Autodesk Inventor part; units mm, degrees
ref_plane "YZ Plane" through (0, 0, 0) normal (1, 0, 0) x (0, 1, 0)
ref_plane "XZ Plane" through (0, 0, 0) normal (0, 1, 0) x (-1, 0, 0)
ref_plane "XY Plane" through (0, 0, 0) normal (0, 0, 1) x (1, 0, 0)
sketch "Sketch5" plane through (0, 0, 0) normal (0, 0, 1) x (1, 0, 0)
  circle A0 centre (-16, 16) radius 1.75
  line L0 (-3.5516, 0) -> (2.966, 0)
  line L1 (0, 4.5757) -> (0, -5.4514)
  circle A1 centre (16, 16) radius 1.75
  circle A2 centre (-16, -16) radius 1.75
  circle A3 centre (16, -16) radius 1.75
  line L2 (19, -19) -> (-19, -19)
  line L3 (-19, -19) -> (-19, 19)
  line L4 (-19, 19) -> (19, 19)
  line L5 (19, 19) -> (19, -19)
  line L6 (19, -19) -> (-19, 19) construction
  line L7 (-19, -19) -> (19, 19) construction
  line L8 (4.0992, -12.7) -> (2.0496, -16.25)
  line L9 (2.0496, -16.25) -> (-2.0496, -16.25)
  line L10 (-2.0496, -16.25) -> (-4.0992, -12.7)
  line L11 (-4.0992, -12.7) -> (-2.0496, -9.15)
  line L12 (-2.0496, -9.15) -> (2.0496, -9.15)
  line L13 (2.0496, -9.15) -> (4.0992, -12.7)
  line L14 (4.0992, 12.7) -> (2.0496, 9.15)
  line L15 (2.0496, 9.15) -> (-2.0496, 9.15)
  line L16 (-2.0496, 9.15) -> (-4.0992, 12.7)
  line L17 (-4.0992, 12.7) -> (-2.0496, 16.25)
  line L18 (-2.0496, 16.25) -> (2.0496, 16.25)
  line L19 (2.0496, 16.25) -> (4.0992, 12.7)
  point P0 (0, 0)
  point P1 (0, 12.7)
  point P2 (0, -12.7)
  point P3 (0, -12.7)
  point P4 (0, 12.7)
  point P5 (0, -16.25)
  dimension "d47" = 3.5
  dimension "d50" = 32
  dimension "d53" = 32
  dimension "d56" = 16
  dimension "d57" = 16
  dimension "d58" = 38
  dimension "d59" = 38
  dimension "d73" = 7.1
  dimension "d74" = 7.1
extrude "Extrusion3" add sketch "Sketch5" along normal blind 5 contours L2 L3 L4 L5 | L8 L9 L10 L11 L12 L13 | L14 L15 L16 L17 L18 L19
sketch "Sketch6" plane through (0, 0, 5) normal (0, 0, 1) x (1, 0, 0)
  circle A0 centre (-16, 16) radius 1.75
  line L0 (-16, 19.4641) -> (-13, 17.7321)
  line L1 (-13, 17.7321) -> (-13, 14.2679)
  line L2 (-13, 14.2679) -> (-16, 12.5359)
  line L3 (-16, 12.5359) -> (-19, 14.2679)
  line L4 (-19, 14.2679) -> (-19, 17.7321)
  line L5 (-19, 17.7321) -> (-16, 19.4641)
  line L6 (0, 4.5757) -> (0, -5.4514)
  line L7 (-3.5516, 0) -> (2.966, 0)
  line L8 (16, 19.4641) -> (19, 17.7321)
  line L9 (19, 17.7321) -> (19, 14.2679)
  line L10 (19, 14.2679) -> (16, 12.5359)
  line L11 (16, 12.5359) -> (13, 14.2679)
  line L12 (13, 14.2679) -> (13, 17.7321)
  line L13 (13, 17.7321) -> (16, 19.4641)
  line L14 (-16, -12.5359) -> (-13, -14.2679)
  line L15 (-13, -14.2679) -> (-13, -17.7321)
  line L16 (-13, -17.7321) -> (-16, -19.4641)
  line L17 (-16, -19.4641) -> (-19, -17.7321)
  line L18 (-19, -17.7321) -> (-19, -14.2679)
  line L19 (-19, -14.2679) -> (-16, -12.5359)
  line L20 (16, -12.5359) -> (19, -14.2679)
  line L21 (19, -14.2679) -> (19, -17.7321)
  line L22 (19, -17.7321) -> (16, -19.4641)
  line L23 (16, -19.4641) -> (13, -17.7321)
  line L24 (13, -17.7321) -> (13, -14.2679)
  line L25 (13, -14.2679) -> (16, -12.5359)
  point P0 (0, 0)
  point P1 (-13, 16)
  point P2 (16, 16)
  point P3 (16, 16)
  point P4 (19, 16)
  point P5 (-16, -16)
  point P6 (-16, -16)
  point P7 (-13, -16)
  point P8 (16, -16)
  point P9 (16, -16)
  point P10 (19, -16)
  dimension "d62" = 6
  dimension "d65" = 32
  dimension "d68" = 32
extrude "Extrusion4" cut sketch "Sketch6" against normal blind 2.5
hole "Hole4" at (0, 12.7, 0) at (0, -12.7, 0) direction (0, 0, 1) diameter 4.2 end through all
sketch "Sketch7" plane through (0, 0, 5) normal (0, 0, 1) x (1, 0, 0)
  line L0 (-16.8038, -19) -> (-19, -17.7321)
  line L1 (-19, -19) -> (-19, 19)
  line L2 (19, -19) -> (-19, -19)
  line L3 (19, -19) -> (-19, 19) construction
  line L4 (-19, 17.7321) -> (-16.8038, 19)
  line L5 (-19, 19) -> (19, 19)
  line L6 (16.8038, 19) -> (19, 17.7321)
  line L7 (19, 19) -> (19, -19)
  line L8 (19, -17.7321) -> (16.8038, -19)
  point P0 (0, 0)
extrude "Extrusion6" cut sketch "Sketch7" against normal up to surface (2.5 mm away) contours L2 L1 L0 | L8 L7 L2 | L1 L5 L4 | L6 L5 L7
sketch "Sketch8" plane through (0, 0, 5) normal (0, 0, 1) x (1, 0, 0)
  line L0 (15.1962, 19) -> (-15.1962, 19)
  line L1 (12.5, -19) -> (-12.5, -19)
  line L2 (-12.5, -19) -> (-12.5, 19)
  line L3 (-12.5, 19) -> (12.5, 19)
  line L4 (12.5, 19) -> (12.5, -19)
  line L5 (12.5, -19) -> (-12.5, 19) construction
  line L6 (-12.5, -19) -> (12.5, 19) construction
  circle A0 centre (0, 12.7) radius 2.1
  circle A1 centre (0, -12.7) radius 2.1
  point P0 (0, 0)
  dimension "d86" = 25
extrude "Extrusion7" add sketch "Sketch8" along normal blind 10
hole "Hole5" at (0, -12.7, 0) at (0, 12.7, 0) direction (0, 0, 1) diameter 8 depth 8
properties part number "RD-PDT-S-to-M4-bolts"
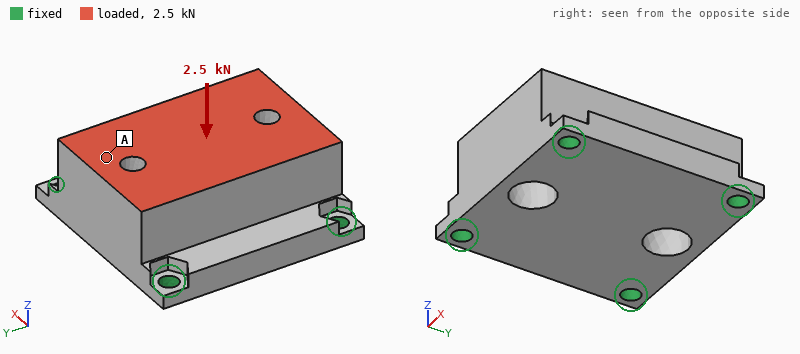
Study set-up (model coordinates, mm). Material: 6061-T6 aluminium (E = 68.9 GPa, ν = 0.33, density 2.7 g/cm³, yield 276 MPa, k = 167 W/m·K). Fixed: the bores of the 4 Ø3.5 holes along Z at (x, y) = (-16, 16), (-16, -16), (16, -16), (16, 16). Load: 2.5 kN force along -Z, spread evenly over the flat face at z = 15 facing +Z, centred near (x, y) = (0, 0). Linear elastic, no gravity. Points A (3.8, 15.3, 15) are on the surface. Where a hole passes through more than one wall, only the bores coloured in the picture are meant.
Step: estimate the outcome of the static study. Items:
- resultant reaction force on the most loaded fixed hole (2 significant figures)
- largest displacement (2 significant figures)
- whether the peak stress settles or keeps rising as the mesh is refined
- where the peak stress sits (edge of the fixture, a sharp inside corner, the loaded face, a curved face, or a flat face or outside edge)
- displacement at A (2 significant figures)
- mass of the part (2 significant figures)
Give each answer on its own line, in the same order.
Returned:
740 N
7.9 µm
keeps rising
edge of the fixture
7.0 µm
41 g
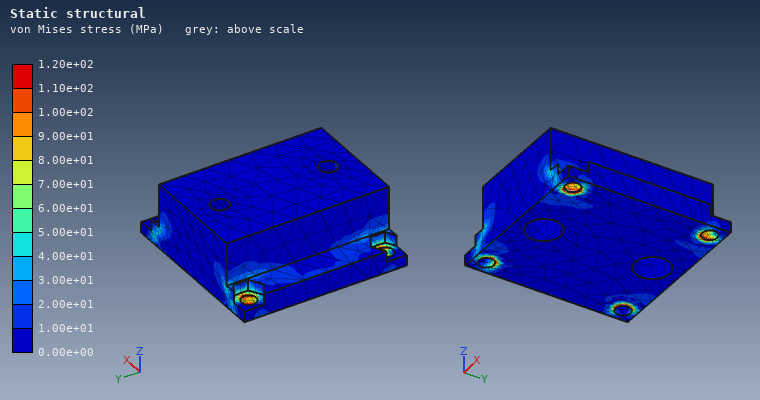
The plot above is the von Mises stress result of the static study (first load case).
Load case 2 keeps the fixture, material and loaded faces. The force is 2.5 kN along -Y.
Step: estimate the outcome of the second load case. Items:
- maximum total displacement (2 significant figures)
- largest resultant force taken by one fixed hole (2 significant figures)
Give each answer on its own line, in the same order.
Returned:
13 µm
930 N
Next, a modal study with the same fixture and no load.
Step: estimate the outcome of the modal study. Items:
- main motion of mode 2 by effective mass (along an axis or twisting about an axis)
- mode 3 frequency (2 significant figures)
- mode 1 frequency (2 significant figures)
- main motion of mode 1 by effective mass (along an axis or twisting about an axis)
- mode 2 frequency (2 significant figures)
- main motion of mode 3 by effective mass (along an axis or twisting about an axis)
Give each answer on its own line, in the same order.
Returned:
along Y
19 kHz
15 kHz
along Z
17 kHz
along X
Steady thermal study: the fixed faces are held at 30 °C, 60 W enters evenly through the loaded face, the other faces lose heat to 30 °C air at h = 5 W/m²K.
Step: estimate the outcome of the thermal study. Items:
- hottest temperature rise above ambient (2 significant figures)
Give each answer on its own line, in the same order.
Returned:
20 K
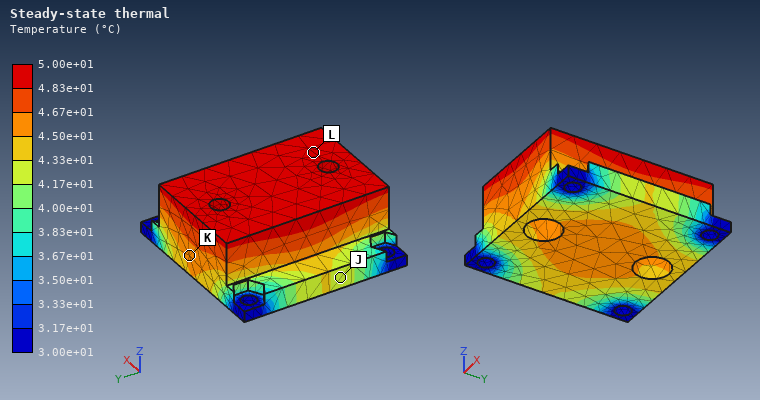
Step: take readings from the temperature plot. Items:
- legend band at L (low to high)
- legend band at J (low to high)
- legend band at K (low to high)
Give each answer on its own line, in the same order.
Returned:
4.83e+01 to 5.00e+01 °C
4.17e+01 to 4.33e+01 °C
4.50e+01 to 4.67e+01 °C
